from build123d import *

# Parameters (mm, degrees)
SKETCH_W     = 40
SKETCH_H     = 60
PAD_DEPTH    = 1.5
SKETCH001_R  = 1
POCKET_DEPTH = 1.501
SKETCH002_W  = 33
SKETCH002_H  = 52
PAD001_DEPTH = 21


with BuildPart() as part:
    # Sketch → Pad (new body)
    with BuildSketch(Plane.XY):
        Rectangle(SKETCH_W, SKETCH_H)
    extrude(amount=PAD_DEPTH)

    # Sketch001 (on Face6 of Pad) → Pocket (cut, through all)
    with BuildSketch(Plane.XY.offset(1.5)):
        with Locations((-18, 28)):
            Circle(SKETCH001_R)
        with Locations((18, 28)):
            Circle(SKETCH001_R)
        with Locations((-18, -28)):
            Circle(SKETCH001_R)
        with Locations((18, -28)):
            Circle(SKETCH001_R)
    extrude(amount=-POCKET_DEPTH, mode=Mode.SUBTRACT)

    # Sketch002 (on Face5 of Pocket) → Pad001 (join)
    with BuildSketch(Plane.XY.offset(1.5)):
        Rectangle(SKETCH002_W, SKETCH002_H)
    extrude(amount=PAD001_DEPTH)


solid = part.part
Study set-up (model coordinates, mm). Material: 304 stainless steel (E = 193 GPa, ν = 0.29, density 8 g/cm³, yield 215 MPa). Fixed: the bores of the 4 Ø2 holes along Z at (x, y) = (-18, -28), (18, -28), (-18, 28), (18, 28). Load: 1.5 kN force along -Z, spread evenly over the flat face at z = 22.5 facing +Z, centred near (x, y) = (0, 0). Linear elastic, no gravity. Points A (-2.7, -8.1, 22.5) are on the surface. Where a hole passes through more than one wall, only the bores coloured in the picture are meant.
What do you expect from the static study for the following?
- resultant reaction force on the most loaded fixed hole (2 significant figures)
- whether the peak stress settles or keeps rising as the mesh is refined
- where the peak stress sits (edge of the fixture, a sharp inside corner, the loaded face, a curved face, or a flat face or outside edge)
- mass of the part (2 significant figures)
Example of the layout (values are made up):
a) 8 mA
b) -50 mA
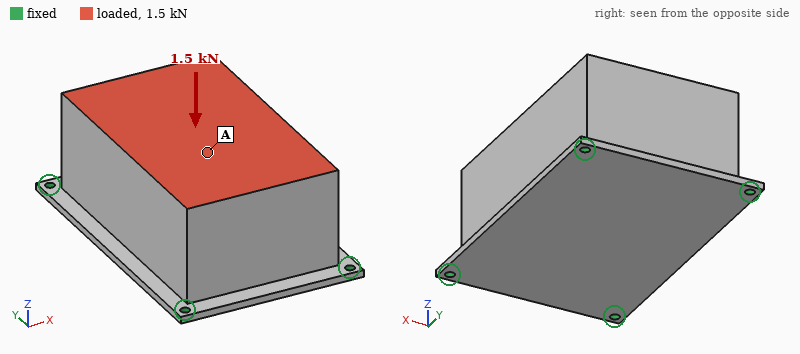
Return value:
a) 430 N
b) keeps rising
c) edge of the fixture
d) 320 g
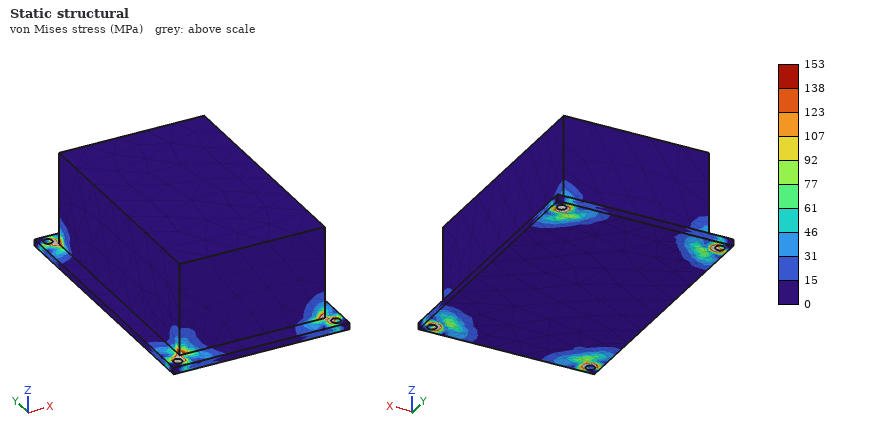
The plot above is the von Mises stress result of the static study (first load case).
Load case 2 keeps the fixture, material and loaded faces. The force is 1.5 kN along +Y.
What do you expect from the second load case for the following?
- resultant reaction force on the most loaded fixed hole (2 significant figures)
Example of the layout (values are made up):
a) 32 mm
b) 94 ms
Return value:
a) 520 N
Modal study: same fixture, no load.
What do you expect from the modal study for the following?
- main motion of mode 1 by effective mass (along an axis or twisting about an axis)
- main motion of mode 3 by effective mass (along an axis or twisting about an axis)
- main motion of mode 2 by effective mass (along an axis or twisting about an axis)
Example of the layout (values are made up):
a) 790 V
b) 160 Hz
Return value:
a) along Z
b) along Y
c) along X
